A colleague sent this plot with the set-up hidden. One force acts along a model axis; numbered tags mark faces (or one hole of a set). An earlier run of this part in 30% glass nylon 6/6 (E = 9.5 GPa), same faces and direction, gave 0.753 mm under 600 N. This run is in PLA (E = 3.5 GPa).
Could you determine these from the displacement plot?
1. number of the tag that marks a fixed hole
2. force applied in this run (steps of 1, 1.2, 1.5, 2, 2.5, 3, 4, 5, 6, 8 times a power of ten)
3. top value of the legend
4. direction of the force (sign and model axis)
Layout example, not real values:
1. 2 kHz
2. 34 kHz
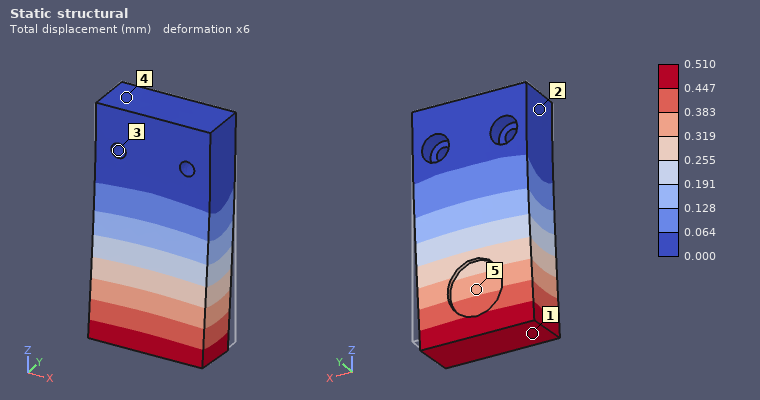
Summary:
1. 3
2. 150 N
3. 0.510 mm
4. -Y
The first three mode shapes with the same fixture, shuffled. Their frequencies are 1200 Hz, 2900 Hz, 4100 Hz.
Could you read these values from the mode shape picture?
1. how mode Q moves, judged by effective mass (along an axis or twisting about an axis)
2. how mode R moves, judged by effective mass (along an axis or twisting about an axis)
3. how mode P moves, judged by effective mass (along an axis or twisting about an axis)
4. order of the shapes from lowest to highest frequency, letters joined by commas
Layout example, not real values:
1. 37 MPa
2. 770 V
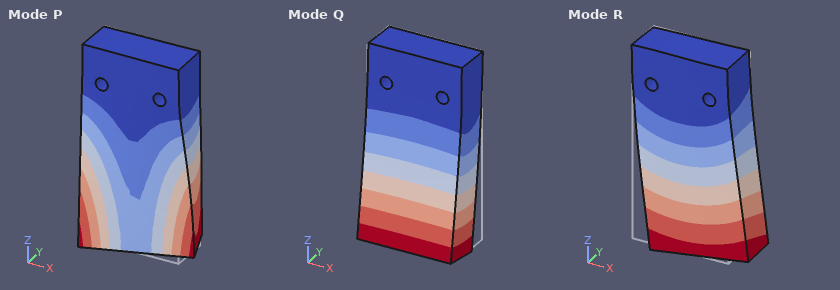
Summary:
1. along Y
2. along X
3. twisting about Z
4. Q, R, P
